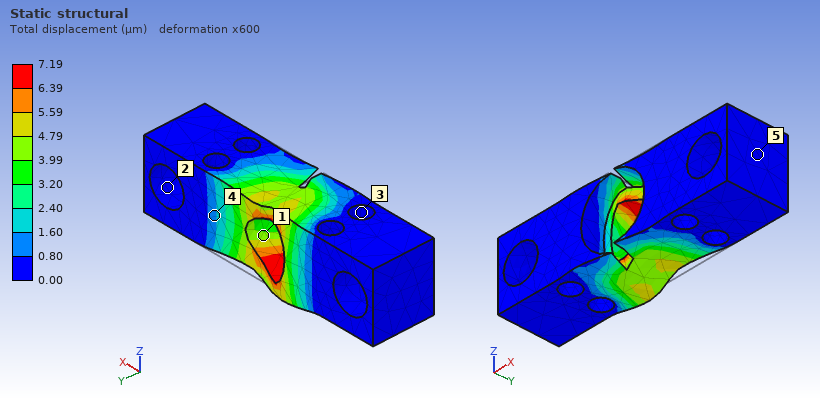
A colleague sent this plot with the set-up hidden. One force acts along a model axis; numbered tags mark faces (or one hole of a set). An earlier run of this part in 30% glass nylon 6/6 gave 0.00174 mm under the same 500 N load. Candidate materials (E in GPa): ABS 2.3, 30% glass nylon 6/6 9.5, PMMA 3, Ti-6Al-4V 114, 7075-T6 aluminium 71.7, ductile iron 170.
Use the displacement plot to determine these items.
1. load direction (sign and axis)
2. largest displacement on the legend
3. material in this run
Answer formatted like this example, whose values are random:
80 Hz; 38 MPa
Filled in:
-X; 7.19 µm; ABS
